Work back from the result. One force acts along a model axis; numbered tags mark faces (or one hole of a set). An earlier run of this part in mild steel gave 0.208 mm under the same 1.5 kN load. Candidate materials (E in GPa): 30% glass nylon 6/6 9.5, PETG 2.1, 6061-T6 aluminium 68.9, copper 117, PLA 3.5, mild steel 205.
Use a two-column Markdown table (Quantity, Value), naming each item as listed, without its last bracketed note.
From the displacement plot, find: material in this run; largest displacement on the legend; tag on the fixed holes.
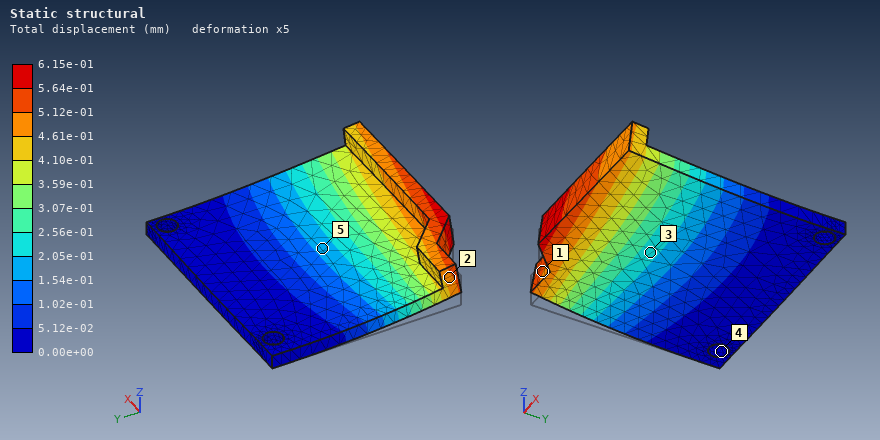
| Quantity | Value |
|---|---|
| material in this run | 6061-T6 aluminium |
| largest displacement on the legend | 6.15e-01 mm |
| tag on the fixed holes | 4 |
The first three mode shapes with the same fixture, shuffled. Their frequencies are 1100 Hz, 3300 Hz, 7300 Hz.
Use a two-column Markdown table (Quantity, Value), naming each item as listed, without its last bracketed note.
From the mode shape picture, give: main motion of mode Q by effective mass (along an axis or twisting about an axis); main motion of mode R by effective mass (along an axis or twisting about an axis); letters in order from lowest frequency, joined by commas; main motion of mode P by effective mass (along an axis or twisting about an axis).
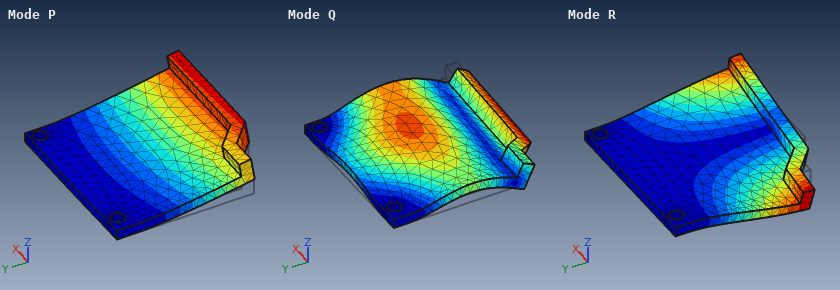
| Quantity | Value |
|---|---|
| main motion of mode Q by effective mass | along Z |
| main motion of mode R by effective mass | twisting about Y |
| letters in order from lowest frequency, joined by commas | P, R, Q |
| main motion of mode P by effective mass | along Z |
